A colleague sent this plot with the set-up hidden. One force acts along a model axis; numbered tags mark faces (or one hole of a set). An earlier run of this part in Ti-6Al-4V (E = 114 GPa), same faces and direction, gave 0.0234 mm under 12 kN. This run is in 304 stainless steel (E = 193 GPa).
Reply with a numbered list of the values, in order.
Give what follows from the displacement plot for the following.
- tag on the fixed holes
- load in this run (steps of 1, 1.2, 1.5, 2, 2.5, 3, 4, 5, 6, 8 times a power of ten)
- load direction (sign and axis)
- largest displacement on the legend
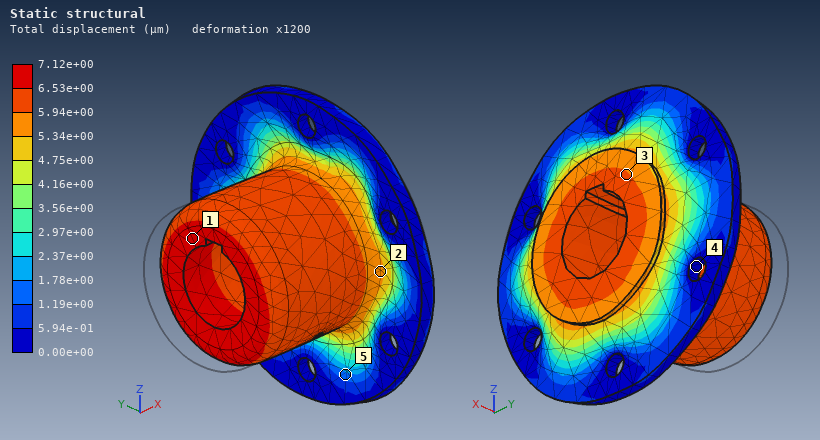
1. 4
2. 6 kN
3. +X
4. 7.12e+00 µm
